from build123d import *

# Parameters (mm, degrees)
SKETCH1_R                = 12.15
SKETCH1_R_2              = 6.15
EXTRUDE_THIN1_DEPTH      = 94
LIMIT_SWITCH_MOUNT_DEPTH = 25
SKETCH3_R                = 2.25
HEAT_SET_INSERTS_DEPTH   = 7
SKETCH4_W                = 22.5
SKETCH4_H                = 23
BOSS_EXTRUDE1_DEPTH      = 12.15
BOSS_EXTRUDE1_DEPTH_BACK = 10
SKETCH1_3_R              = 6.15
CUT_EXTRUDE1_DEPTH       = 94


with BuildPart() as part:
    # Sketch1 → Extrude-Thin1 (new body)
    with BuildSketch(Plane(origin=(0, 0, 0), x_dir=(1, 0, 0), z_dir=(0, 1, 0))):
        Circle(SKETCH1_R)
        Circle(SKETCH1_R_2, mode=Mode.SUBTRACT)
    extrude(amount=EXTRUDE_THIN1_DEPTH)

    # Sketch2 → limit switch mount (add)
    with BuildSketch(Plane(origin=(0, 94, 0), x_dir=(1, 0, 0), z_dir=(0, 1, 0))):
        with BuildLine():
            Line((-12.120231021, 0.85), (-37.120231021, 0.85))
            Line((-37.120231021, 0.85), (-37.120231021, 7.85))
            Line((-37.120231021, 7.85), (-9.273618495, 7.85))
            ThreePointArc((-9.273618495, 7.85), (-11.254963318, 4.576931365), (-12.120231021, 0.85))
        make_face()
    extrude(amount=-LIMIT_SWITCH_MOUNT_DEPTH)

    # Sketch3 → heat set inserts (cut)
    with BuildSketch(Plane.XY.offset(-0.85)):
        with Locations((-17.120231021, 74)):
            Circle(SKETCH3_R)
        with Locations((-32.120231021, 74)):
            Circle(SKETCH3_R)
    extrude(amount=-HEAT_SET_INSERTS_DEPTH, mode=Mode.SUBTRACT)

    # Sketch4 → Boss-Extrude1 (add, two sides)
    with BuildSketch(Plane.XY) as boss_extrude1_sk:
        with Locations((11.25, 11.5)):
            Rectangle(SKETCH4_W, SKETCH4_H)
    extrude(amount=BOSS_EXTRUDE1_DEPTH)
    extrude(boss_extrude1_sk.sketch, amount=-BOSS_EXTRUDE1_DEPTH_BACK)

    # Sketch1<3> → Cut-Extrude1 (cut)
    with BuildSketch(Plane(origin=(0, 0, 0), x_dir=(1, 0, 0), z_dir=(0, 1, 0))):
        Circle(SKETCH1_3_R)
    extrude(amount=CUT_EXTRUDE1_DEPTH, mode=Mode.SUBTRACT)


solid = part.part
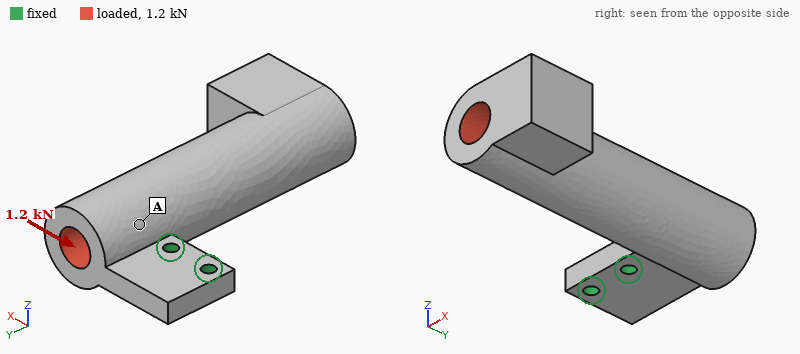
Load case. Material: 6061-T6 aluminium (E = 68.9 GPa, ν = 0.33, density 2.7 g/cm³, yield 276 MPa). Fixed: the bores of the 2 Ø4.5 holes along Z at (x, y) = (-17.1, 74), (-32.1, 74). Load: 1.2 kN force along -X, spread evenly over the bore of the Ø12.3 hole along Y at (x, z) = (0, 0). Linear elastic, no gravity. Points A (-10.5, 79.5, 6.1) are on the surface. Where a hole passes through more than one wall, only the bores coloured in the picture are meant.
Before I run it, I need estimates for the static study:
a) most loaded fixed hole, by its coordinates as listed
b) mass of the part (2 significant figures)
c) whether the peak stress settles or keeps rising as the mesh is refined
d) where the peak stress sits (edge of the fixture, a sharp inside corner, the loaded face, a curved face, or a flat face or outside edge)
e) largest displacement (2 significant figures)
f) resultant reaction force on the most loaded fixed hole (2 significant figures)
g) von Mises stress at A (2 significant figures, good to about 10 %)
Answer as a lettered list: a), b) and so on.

a) (-17.1, 74)
b) 120 g
c) keeps rising
d) edge of the fixture
e) 0.23 mm
f) 2.5 kN
g) 12 MPa
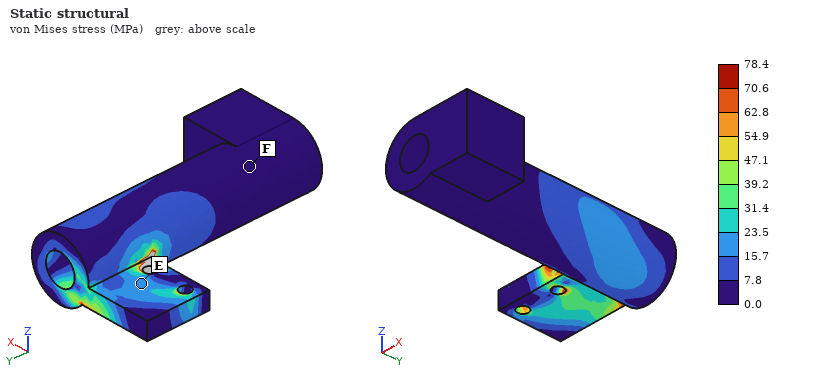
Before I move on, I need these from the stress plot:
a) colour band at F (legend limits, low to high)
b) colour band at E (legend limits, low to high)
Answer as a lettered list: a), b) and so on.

a) 0.0 to 7.8 MPa
b) 15.7 to 23.5 MPa
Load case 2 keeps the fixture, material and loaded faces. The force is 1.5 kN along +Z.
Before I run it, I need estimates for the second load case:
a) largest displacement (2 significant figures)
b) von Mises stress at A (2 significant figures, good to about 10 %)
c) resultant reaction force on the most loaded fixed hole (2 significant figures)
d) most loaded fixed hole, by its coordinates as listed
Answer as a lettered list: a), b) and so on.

a) 0.64 mm
b) 37 MPa
c) 2.0 kN
d) (-17.1, 74)
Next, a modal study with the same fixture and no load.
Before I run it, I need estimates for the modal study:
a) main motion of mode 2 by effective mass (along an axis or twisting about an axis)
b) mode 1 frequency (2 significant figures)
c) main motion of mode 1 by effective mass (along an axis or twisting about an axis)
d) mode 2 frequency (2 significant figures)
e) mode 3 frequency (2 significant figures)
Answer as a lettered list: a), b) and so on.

a) along X
b) 820 Hz
c) along Z
d) 1200 Hz
e) 2500 Hz
